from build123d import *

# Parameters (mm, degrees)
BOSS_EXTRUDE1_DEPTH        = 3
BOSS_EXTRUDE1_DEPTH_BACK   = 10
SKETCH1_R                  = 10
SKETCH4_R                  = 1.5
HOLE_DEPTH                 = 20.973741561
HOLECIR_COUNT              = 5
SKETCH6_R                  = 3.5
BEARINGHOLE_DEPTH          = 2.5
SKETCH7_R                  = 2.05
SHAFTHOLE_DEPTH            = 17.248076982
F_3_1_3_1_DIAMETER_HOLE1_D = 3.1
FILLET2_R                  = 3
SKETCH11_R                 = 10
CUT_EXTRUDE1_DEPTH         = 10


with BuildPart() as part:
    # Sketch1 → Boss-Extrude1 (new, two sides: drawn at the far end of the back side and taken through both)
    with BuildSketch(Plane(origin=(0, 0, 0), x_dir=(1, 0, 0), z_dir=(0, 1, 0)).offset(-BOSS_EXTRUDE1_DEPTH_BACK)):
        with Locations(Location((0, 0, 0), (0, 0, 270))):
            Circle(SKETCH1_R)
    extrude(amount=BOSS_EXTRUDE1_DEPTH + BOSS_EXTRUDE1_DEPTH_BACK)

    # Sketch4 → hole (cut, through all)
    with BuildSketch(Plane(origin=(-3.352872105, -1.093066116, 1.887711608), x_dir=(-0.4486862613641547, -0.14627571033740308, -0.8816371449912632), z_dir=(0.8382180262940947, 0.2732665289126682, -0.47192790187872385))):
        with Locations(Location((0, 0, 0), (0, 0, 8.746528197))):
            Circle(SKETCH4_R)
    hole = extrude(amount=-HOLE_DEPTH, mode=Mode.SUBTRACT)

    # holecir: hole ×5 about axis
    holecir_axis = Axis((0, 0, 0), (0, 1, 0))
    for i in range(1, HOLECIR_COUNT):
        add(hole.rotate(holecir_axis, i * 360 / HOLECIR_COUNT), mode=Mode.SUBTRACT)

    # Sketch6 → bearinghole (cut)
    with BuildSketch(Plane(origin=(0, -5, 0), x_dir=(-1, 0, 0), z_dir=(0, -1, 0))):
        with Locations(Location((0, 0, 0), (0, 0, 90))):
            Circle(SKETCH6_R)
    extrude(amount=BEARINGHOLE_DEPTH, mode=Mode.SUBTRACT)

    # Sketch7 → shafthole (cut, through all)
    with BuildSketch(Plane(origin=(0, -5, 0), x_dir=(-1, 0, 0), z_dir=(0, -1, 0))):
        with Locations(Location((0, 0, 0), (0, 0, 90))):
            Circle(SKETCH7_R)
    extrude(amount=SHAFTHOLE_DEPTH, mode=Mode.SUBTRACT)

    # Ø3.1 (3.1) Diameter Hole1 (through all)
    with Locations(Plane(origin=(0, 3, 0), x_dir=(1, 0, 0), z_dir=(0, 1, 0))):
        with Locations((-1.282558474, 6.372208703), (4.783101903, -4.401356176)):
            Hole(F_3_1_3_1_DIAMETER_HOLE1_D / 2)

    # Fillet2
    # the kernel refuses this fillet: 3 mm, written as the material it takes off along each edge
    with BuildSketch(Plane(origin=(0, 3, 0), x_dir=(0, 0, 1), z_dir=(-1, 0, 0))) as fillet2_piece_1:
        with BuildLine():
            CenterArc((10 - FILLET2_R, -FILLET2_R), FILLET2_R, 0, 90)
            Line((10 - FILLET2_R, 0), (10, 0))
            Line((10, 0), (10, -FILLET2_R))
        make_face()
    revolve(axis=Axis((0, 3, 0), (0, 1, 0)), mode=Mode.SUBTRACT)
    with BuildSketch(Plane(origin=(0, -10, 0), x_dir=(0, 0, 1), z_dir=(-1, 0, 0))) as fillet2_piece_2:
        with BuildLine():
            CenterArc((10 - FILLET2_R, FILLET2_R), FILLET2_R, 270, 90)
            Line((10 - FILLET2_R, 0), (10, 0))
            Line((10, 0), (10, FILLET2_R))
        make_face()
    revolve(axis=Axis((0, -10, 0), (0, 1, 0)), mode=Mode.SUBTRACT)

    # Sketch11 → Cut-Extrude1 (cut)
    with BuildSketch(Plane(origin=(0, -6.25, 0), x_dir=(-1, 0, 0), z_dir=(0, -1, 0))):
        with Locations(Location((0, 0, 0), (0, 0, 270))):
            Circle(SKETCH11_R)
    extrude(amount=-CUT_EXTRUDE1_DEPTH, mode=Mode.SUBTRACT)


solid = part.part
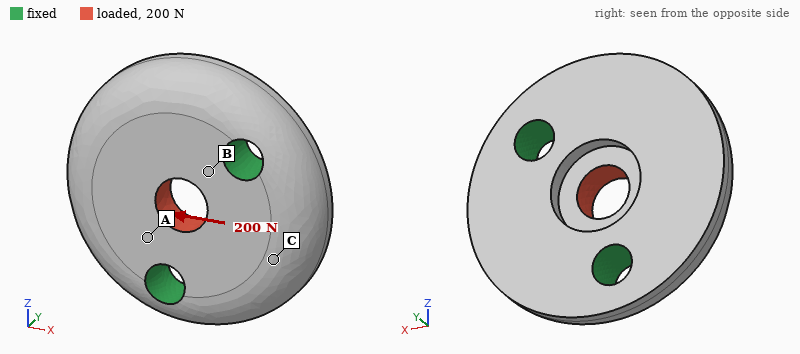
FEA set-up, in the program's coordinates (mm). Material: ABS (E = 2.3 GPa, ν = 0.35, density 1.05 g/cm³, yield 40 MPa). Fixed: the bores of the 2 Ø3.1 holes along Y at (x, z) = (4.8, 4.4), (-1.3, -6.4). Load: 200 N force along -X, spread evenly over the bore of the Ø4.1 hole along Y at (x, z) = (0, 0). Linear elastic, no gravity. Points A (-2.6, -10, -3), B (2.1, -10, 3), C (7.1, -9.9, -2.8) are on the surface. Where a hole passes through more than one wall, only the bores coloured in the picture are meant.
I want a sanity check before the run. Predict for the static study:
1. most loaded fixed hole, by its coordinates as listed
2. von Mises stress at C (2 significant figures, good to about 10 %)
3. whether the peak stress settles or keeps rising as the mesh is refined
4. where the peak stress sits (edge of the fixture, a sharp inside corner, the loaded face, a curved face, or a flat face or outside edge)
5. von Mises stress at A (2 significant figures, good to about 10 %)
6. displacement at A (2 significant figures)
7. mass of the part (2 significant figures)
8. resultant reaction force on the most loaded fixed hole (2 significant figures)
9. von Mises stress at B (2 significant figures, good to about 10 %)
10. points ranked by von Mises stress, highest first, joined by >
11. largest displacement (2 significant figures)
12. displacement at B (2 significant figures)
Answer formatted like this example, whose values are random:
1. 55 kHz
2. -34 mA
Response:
1. (4.8, 4.4)
2. 1.6 MPa
3. keeps rising
4. edge of the fixture
5. 5.2 MPa
6. 11 µm
7. 0.97 g
8. 110 N
9. 7.5 MPa
10. B > A > C
11. 22 µm
12. 6.6 µm
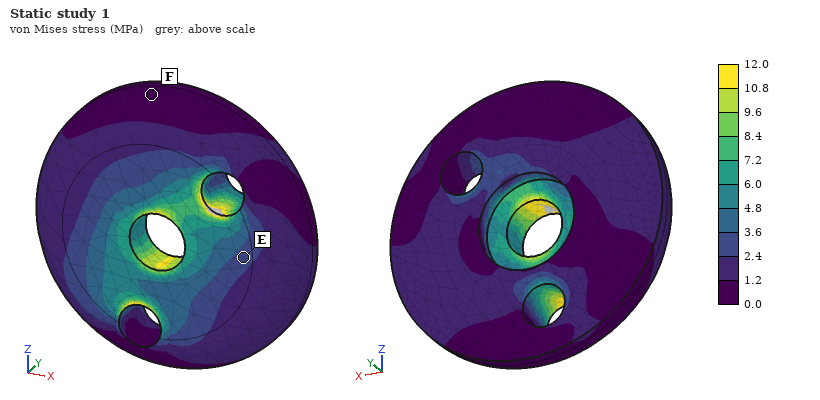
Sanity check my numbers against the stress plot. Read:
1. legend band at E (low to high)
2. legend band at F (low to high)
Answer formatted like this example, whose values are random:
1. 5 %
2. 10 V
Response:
1. 2.4 to 3.6 MPa
2. 0.0 to 1.2 MPa
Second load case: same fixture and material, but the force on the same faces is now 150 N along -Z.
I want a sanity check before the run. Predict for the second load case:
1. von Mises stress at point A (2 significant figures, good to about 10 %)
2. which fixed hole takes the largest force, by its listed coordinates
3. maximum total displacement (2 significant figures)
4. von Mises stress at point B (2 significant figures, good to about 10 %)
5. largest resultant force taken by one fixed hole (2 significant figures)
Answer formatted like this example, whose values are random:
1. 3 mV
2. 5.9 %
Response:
1. 4.7 MPa
2. (-1.3, -6.4)
3. 16 µm
4. 4.8 MPa
5. 85 N
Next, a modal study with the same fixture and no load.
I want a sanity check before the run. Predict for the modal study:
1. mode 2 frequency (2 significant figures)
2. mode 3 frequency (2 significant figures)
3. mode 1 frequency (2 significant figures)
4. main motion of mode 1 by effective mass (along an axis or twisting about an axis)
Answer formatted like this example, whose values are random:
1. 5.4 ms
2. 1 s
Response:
1. 16 kHz
2. 16 kHz
3. 7500 Hz
4. along Y
